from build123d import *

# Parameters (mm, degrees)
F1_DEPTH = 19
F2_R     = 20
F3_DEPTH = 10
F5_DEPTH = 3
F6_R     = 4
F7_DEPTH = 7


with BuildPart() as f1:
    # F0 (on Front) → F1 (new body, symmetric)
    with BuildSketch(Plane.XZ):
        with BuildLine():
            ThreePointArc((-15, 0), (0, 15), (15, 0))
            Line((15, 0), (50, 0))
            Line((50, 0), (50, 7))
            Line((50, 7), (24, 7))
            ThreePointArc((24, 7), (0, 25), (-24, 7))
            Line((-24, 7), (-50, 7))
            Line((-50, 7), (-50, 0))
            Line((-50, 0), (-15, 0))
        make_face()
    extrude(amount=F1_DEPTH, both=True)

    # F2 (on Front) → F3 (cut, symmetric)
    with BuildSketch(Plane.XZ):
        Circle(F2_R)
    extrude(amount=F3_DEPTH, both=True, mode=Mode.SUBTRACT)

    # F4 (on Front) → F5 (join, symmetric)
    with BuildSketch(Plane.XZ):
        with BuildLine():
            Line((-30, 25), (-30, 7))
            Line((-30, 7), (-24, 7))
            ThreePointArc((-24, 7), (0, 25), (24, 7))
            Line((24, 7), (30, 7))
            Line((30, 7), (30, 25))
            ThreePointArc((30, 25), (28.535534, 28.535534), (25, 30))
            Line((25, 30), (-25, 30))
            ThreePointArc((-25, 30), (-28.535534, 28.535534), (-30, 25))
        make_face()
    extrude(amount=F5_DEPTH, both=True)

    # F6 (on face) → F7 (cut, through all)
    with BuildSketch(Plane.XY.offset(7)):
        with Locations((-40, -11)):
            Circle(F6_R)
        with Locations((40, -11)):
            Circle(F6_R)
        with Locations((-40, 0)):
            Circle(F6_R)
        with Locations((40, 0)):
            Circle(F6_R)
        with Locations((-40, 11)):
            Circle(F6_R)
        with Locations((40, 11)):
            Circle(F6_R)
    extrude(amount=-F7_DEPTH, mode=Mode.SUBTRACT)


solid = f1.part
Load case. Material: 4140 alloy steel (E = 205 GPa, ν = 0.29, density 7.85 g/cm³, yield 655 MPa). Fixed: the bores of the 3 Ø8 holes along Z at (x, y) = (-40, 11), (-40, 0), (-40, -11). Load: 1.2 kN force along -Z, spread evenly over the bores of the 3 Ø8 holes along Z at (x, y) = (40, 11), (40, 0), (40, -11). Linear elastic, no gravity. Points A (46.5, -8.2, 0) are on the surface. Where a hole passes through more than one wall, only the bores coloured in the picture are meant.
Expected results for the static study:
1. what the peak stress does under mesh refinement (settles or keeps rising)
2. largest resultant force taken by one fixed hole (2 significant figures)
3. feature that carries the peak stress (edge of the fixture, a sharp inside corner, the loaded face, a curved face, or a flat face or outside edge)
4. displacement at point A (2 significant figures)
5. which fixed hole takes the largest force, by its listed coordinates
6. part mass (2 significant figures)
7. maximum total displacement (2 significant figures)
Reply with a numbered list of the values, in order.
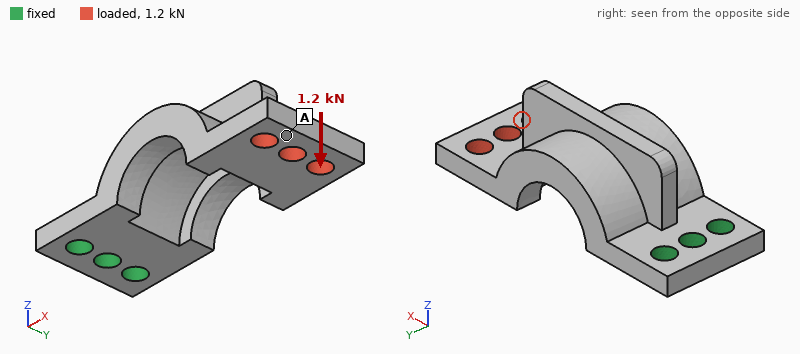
1. keeps rising
2. 1.5 kN
3. edge of the fixture
4. 0.60 mm
5. (-40, 0)
6. 270 g
7. 0.63 mm
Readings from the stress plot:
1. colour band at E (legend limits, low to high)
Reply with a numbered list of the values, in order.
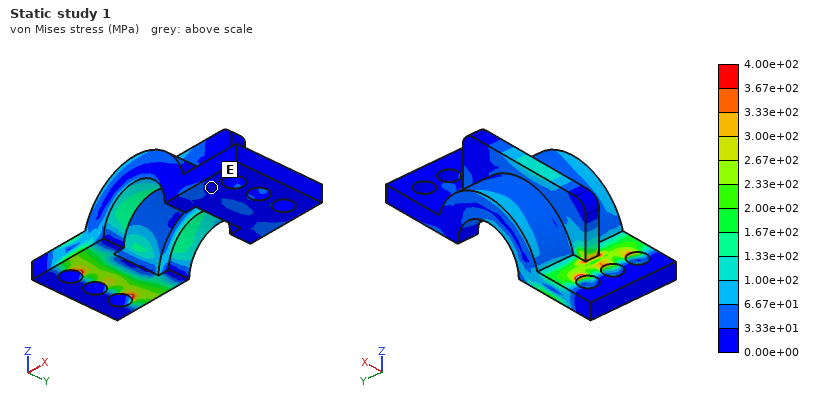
1. 0.00e+00 to 3.33e+01 MPa
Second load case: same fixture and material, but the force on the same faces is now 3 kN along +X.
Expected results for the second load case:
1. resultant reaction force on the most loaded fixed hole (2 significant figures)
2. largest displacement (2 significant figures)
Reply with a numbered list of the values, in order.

1. 1.3 kN
2. 0.17 mm
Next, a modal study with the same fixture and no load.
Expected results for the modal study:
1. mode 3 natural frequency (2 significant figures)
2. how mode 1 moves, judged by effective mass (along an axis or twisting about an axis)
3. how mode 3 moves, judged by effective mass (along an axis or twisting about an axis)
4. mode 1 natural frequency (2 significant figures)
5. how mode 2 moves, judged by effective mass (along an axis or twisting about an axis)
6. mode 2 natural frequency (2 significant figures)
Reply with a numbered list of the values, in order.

1. 3600 Hz
2. along Z
3. along X
4. 850 Hz
5. along Y
6. 1600 Hz
